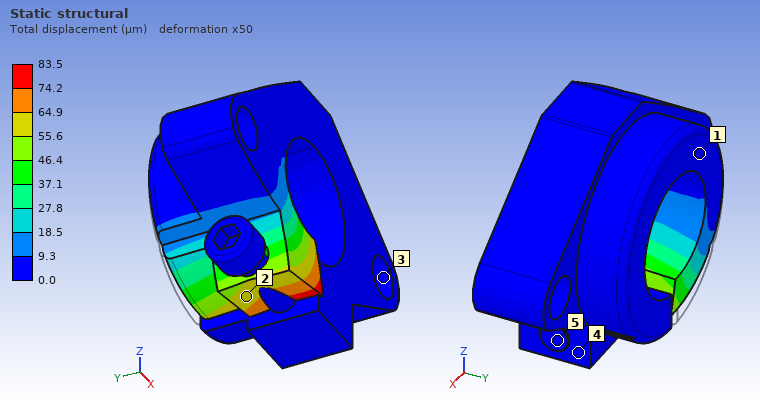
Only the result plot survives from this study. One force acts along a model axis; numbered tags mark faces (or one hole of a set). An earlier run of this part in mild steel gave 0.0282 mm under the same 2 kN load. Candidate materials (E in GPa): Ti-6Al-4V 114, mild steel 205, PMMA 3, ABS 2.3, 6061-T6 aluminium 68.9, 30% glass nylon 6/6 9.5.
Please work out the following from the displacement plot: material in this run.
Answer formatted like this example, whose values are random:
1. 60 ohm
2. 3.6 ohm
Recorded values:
1. 6061-T6 aluminium
